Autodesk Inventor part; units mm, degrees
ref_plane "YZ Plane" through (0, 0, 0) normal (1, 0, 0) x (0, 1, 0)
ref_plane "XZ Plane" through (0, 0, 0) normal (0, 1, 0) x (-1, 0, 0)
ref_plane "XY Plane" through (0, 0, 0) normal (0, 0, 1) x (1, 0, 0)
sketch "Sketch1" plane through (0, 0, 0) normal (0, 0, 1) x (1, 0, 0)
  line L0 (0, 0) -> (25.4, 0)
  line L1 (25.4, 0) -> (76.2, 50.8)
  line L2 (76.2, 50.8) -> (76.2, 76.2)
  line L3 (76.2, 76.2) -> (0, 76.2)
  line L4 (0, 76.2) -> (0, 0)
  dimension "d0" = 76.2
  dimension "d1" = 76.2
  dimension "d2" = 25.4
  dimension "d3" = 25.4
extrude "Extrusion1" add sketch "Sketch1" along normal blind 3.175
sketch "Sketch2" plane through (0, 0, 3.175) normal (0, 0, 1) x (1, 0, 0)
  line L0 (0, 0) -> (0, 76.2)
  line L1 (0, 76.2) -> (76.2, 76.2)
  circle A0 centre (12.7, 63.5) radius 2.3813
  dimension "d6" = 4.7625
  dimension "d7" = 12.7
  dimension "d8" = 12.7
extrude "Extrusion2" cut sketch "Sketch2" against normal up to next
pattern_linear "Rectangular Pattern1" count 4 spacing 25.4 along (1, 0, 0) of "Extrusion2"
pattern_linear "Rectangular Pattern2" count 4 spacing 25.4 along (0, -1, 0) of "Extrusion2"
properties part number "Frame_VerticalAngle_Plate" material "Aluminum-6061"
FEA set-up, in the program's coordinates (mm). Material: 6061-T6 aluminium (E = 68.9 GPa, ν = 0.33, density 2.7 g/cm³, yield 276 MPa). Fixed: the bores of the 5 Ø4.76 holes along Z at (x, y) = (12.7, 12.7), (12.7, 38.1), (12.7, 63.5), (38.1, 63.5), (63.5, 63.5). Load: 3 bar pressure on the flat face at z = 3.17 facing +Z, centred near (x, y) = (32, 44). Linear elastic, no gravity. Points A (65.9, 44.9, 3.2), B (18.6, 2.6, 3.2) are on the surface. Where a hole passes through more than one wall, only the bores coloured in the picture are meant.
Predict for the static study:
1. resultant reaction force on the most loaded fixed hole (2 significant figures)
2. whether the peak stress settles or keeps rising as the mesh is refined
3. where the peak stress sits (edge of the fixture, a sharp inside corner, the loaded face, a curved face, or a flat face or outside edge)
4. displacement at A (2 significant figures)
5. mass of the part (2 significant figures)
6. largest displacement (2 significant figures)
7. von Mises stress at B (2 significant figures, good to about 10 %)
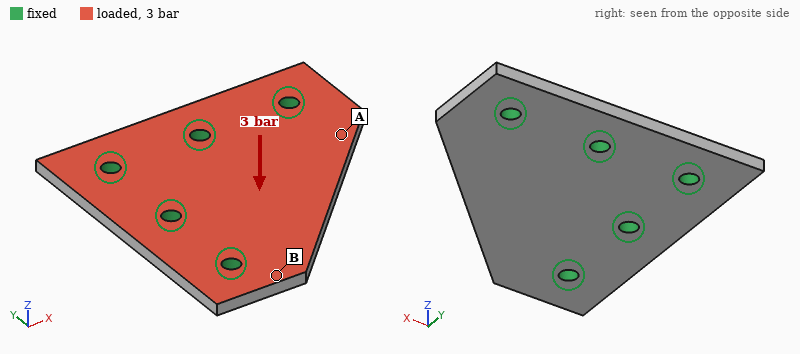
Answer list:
310 N
keeps rising
edge of the fixture
0.055 mm
38 g
0.12 mm
26 MPa
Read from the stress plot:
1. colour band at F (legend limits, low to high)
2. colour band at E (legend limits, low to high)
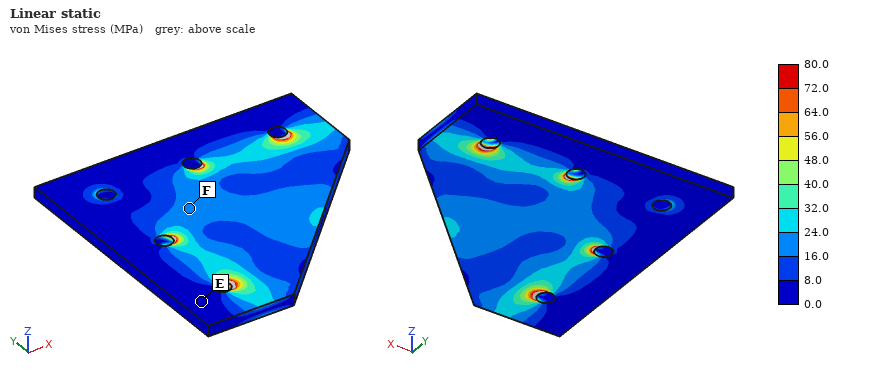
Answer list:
16.0 to 24.0 MPa
0.0 to 8.0 MPa
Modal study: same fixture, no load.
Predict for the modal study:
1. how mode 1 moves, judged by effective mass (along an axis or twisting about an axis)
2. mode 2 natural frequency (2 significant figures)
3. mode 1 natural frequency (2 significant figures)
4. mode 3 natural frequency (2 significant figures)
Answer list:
along Z
7600 Hz
3700 Hz
11 kHz
